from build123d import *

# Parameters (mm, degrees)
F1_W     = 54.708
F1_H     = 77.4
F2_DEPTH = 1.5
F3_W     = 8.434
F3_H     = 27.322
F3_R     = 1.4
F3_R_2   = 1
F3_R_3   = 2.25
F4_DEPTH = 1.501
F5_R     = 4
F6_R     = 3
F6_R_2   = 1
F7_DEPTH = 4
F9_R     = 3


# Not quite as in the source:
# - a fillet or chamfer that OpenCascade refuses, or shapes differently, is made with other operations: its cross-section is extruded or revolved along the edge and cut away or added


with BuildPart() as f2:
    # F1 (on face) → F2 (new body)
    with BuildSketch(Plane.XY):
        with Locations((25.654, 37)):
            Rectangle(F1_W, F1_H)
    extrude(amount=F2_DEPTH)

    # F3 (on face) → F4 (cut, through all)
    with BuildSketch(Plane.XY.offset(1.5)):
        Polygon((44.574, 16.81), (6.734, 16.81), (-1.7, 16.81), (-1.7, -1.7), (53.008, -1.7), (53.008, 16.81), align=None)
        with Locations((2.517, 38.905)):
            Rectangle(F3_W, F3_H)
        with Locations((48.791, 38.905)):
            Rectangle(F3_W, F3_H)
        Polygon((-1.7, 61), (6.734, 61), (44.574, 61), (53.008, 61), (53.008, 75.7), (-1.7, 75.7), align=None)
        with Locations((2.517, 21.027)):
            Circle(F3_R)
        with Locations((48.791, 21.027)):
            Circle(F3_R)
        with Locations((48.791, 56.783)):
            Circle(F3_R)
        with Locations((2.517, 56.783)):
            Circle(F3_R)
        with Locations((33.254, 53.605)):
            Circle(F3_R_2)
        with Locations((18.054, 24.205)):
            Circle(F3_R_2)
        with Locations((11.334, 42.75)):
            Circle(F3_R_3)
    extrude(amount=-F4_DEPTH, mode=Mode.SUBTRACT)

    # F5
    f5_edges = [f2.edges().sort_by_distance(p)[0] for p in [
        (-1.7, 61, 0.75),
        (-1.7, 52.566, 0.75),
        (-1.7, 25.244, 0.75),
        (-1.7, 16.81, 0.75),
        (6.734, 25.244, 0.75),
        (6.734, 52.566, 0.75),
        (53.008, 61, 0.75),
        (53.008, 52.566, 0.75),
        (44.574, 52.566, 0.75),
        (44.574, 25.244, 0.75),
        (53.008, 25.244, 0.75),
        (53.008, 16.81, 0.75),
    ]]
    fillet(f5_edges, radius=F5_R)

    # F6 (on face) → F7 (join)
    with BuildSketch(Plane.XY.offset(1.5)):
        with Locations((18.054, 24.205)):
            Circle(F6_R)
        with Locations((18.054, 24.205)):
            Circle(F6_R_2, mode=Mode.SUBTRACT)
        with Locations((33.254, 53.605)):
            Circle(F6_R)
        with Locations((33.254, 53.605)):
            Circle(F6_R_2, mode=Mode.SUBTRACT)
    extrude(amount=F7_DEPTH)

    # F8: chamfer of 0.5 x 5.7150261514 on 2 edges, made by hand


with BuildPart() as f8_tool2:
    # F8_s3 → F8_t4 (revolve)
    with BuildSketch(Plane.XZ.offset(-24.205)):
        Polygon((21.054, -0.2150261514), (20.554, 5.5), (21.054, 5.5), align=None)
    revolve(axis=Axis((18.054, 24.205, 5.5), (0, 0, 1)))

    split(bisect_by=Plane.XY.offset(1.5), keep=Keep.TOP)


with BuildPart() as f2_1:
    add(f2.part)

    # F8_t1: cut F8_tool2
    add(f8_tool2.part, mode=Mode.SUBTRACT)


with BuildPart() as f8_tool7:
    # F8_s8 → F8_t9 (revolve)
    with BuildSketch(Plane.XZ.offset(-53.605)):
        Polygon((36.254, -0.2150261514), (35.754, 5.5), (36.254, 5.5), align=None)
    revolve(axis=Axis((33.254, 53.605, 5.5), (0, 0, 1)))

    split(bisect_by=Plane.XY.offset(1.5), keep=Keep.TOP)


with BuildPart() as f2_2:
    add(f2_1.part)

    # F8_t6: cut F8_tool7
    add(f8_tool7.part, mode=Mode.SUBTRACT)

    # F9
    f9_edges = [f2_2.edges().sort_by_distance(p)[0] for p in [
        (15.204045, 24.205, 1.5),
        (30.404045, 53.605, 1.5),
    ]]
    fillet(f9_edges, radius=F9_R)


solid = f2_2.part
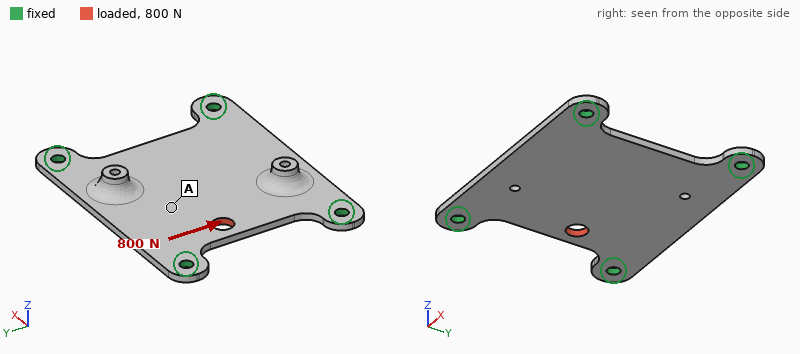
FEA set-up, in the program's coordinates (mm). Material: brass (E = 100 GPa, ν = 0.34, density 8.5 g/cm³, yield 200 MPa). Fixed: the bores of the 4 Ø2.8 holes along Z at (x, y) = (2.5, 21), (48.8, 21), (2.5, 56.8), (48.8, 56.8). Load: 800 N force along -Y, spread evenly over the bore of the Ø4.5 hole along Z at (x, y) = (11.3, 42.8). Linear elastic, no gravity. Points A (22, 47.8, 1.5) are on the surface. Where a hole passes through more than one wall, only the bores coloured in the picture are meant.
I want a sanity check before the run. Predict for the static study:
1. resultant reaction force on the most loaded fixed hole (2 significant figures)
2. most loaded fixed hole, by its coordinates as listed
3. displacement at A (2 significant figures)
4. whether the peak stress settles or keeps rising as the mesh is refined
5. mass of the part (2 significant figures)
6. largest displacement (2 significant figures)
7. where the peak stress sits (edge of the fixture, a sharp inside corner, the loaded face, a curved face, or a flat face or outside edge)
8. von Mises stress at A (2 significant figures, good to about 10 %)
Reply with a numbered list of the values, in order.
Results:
1. 320 N
2. (2.5, 56.8)
3. 5.8 µm
4. keeps rising
5. 26 g
6. 9.2 µm
7. edge of the fixture
8. 12 MPa
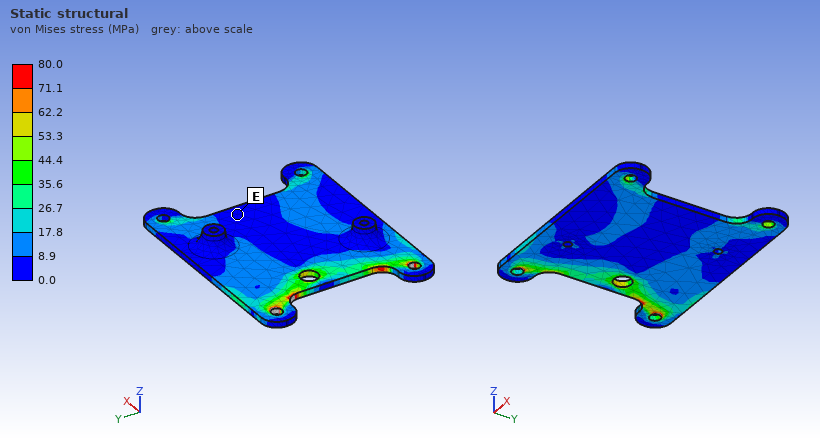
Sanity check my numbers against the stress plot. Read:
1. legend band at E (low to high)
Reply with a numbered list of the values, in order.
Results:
1. 0.0 to 8.9 MPa
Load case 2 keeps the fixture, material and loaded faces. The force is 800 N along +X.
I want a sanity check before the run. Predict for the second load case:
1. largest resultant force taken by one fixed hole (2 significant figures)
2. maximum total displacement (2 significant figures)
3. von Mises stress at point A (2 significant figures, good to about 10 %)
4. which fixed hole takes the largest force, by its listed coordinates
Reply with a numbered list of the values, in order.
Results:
1. 300 N
2. 10 µm
3. 20 MPa
4. (2.5, 56.8)
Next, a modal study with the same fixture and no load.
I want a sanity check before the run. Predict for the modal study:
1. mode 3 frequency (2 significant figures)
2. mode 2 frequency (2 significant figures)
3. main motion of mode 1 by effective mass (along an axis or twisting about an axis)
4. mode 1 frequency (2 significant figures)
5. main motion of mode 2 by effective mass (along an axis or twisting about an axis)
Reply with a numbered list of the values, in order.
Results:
1. 4100 Hz
2. 3000 Hz
3. along Z
4. 1900 Hz
5. twisting about X
